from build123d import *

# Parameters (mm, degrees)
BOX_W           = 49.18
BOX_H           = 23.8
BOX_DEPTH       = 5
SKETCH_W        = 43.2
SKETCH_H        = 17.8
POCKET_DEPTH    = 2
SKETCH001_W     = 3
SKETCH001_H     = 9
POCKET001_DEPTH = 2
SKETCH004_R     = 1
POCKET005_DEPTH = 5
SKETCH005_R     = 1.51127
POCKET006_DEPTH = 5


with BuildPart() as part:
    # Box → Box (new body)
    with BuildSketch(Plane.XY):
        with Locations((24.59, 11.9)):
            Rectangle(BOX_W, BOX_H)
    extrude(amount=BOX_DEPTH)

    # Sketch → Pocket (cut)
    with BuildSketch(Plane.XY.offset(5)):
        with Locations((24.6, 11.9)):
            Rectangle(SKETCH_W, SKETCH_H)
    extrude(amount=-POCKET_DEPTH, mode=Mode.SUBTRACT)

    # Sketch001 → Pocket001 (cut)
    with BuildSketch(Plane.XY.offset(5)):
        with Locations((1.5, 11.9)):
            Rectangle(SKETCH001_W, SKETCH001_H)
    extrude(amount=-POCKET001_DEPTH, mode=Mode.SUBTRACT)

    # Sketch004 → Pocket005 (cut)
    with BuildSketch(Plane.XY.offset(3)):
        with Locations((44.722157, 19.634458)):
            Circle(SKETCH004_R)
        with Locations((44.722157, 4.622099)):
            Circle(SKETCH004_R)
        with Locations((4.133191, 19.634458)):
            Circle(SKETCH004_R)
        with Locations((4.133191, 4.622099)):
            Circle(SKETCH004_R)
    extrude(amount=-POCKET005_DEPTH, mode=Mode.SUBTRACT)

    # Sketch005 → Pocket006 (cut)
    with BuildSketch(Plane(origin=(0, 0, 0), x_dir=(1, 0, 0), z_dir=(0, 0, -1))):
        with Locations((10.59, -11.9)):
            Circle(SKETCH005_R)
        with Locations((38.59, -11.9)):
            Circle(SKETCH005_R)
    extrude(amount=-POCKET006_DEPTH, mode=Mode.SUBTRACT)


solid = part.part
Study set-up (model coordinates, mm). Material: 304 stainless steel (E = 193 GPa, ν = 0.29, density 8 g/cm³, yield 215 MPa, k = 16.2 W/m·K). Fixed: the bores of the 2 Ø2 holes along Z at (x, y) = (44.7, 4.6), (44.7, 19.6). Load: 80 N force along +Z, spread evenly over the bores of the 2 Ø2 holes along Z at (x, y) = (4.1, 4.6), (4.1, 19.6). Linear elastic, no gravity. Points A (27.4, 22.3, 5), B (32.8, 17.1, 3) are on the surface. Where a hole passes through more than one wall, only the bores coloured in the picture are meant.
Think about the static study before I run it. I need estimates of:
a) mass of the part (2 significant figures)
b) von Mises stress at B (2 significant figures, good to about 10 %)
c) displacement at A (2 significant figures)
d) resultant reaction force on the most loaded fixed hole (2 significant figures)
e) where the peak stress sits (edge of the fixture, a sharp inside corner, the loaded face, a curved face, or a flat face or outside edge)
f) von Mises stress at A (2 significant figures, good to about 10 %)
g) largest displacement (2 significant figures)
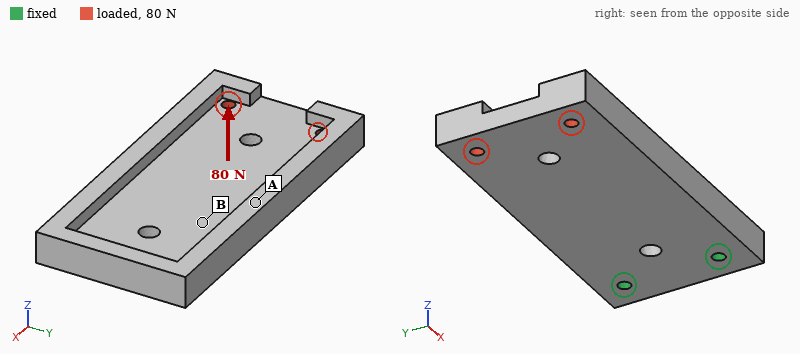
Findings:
33 g
21 MPa
0.027 mm
50 N
edge of the fixture
48 MPa
0.11 mm
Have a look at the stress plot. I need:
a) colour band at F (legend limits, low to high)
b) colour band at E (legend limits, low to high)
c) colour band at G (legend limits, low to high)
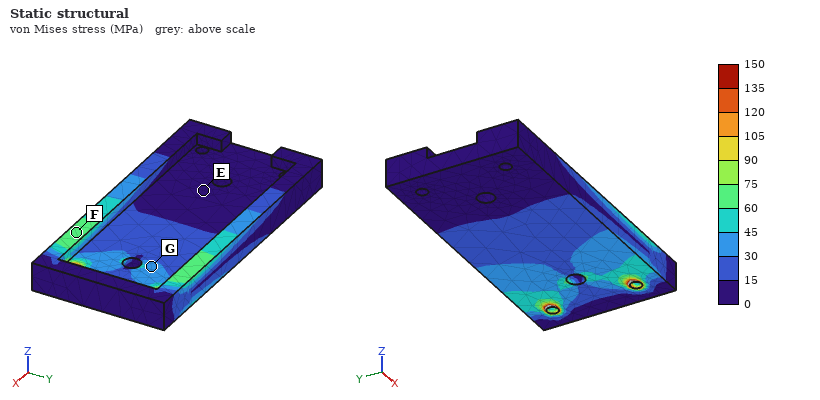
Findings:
60 to 75 MPa
0 to 15 MPa
30 to 45 MPa
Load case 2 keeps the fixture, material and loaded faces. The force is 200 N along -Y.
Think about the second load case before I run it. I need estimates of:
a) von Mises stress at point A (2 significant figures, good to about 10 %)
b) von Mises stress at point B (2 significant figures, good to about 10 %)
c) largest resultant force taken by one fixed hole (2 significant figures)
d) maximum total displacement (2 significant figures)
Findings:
9.0 MPa
9.4 MPa
520 N
10 µm
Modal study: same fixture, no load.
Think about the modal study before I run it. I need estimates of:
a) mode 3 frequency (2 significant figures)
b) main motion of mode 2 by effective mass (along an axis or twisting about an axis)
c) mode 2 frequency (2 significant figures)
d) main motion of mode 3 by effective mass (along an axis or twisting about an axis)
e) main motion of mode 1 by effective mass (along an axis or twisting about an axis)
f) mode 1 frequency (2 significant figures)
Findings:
7200 Hz
twisting about X
4500 Hz
along Y
along Z
1400 Hz
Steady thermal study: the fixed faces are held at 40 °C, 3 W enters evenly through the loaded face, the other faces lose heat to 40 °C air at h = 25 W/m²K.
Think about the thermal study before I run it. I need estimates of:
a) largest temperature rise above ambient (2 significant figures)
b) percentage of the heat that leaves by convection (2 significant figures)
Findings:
56 K
62 %
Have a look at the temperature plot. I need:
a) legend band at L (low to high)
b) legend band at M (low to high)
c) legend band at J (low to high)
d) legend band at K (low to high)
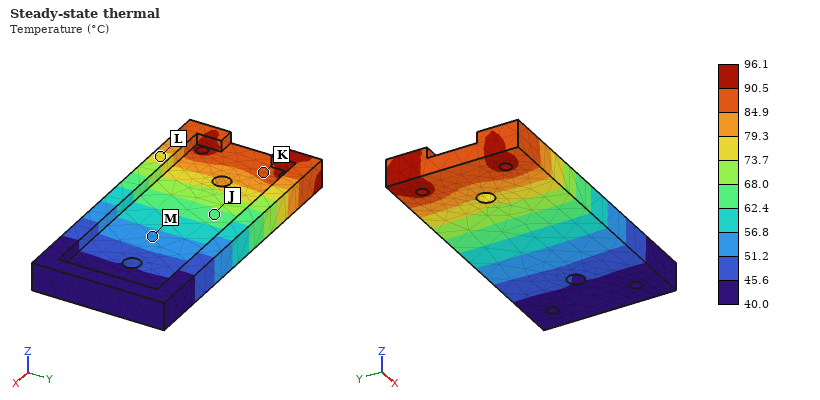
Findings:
73.7 to 79.3 °C
51.2 to 56.8 °C
62.4 to 68.0 °C
84.9 to 90.5 °C
